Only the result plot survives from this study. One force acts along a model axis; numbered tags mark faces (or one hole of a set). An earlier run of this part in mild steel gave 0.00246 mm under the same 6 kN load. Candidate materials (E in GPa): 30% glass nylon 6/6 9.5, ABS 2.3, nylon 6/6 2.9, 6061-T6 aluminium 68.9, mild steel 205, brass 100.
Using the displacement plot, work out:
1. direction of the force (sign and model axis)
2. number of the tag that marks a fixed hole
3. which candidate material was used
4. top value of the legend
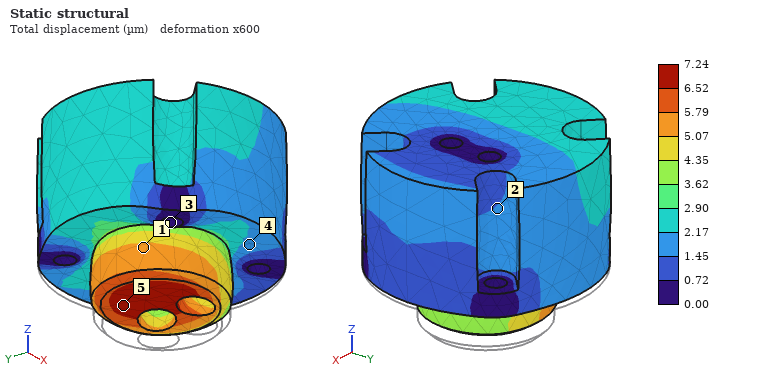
+Z
3
6061-T6 aluminium
7.24 µm
